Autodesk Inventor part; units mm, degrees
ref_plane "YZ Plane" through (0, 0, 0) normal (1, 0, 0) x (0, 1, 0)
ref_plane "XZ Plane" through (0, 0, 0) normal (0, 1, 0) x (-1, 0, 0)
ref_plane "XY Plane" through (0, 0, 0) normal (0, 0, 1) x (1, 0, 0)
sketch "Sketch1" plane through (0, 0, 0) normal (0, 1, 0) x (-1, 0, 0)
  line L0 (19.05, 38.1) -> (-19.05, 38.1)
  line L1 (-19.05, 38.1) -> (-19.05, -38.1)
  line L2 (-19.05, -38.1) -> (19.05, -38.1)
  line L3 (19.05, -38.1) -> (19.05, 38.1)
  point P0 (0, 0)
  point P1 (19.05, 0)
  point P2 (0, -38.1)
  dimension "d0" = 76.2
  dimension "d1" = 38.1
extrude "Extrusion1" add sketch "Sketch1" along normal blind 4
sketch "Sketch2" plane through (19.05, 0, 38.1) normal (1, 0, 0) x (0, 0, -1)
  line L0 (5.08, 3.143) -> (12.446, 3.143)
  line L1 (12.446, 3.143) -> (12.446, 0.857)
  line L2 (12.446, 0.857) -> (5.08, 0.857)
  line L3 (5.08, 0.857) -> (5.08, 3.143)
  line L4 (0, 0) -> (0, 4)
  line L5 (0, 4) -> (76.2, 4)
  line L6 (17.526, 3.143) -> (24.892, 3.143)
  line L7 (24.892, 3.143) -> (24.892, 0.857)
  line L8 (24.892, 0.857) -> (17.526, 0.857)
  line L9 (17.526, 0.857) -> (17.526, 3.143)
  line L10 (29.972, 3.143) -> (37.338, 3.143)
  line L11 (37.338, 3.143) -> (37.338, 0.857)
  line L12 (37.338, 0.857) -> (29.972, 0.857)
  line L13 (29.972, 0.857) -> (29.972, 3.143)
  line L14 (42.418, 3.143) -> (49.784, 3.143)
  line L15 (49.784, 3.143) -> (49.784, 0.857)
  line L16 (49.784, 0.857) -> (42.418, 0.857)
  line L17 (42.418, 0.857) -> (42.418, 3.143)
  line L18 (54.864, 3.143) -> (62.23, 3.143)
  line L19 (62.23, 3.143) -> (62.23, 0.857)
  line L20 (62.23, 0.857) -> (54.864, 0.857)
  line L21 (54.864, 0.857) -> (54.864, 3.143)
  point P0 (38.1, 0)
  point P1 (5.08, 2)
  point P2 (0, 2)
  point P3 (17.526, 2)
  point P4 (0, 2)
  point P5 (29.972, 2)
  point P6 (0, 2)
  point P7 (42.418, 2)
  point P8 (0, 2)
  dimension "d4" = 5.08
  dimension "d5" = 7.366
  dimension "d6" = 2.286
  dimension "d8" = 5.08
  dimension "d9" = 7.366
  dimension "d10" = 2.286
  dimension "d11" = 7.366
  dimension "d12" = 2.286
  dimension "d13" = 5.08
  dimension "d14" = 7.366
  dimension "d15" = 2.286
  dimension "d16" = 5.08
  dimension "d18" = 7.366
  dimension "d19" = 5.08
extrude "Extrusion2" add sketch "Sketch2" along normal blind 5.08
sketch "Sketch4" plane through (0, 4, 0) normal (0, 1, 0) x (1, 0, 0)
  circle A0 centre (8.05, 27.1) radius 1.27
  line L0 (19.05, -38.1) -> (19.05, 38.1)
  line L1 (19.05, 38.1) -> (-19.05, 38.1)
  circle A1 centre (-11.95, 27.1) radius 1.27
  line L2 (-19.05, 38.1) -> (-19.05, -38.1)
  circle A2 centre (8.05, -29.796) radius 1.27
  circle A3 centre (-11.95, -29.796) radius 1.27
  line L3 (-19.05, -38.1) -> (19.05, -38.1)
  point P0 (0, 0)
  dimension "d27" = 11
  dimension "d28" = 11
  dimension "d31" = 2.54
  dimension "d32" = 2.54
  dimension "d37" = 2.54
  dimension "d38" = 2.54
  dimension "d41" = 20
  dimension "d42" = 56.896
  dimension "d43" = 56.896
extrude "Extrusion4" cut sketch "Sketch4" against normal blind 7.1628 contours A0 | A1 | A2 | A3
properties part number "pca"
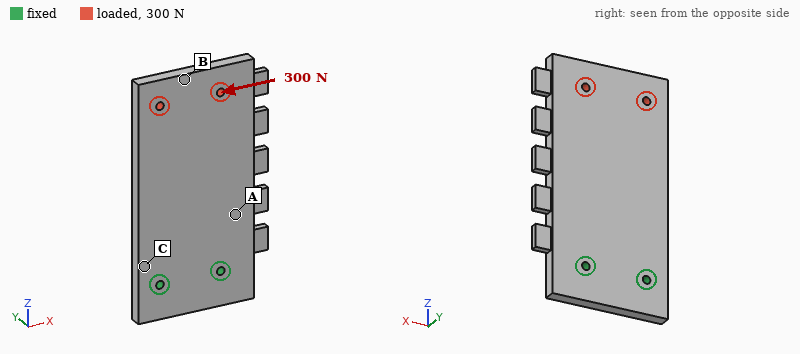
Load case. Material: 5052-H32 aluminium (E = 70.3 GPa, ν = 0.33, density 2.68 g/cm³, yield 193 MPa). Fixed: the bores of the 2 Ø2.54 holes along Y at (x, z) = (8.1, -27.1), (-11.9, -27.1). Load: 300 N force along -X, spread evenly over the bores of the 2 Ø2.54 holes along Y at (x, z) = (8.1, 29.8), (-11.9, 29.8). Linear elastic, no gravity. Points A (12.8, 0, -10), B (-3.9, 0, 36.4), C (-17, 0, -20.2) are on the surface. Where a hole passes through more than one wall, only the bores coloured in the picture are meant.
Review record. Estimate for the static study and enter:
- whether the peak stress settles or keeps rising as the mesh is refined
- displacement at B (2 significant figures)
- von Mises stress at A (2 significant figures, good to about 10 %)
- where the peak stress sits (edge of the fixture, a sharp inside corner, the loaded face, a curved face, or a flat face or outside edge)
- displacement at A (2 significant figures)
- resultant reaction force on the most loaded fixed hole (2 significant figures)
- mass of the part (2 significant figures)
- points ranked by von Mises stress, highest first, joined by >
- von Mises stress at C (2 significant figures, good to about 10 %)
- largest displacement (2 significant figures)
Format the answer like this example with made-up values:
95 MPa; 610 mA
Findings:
keeps rising; 30 µm; 8.2 MPa; edge of the fixture; 7.4 µm; 820 N; 32 g; C > A > B; 13 MPa; 32 µm
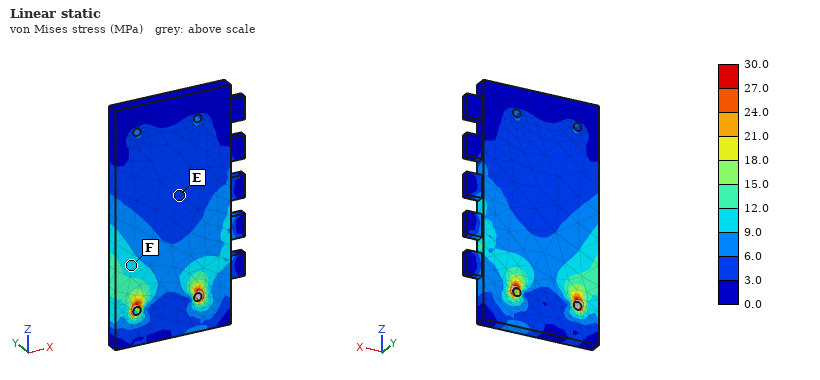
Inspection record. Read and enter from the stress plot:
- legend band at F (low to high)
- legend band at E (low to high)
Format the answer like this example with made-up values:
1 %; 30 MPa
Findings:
9.0 to 12.0 MPa; 3.0 to 6.0 MPa
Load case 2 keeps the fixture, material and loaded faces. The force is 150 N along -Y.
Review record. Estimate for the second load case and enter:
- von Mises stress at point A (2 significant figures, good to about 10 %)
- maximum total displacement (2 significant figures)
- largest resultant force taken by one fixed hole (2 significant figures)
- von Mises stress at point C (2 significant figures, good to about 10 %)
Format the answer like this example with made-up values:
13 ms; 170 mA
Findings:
56 MPa; 0.83 mm; 77 N; 76 MPa
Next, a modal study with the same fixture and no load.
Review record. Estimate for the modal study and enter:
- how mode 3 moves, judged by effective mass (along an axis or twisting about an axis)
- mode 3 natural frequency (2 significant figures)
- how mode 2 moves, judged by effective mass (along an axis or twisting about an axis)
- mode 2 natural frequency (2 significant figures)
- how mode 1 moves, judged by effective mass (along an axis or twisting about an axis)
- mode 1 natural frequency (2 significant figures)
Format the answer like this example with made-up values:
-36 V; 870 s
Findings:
along Y; 4500 Hz; twisting about Z; 2600 Hz; along Y; 740 Hz
